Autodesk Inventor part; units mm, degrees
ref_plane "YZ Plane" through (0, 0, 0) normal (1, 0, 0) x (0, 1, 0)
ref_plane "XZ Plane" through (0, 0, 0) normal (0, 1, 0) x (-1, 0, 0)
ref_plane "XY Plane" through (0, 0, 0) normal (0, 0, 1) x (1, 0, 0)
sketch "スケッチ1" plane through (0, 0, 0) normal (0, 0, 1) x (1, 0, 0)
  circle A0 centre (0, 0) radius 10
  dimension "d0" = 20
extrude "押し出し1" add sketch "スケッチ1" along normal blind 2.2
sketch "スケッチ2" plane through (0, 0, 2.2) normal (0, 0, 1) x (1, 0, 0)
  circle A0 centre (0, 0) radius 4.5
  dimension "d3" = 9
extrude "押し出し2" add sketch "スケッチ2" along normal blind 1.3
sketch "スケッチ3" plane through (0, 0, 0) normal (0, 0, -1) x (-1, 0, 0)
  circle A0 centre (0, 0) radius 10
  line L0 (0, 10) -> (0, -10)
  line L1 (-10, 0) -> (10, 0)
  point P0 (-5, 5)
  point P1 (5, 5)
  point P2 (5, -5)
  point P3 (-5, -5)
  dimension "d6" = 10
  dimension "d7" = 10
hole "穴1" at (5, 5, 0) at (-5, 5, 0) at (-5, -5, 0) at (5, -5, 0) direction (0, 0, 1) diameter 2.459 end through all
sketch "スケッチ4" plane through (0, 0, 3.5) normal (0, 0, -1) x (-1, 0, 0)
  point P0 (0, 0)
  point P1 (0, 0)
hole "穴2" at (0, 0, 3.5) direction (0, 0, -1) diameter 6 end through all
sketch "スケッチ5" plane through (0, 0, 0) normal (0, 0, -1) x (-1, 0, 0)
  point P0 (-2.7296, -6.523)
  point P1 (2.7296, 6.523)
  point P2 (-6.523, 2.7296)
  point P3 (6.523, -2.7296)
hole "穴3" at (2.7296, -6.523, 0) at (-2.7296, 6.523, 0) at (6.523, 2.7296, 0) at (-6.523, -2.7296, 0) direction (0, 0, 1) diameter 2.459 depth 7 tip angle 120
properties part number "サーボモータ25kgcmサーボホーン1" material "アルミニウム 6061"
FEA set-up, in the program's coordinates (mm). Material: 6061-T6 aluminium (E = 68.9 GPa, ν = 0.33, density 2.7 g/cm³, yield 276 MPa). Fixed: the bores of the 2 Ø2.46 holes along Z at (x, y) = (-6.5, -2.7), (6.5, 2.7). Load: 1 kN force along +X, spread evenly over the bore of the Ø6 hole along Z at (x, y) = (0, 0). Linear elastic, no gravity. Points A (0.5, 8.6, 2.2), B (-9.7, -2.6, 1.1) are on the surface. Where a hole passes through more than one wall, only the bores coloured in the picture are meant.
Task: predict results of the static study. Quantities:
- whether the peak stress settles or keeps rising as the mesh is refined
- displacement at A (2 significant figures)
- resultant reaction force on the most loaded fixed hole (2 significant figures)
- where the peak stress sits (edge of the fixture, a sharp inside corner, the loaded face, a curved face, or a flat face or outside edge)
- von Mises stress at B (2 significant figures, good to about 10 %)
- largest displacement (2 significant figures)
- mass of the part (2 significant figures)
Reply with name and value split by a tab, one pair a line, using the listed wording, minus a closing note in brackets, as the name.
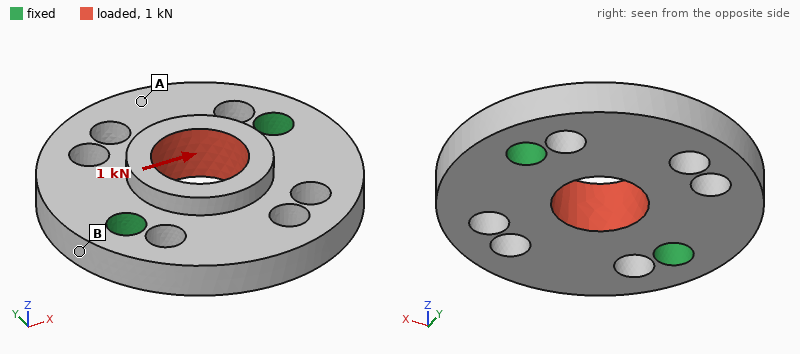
whether the peak stress settles or keeps rising as the mesh is refined	keeps rising
displacement at A	3.7 µm
resultant reaction force on the most loaded fixed hole	500 N
where the peak stress sits	edge of the fixture
von Mises stress at B	20 MPa
largest displacement	5.4 µm
mass of the part	1.6 g
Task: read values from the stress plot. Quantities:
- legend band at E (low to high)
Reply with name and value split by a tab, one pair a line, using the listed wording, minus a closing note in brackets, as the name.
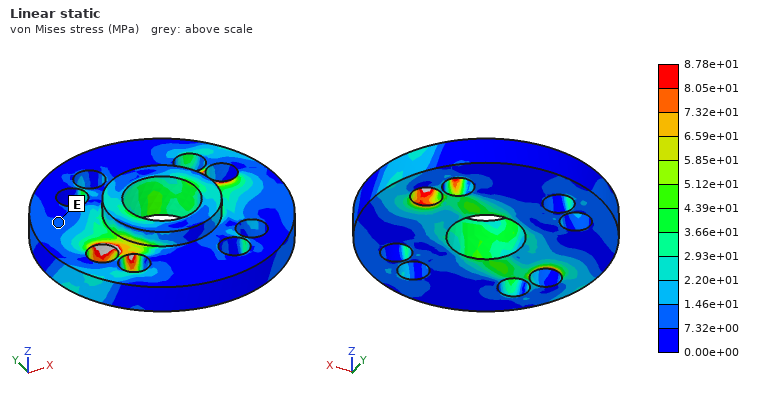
legend band at E	7.32e+00 to 1.46e+01 MPa
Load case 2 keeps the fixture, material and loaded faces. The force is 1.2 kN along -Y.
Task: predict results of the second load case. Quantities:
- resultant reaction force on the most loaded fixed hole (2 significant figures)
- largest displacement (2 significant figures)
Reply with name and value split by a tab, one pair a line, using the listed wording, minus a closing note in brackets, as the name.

resultant reaction force on the most loaded fixed hole	600 N
largest displacement	15 µm
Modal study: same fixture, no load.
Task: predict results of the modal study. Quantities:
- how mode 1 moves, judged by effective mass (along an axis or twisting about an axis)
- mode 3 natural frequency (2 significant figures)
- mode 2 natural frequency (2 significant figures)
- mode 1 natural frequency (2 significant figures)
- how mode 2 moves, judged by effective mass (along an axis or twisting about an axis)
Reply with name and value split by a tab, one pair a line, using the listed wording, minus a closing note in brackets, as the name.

how mode 1 moves, judged by effective mass	twisting about X
mode 3 natural frequency	43 kHz
mode 2 natural frequency	23 kHz
mode 1 natural frequency	18 kHz
how mode 2 moves, judged by effective mass	along Z
